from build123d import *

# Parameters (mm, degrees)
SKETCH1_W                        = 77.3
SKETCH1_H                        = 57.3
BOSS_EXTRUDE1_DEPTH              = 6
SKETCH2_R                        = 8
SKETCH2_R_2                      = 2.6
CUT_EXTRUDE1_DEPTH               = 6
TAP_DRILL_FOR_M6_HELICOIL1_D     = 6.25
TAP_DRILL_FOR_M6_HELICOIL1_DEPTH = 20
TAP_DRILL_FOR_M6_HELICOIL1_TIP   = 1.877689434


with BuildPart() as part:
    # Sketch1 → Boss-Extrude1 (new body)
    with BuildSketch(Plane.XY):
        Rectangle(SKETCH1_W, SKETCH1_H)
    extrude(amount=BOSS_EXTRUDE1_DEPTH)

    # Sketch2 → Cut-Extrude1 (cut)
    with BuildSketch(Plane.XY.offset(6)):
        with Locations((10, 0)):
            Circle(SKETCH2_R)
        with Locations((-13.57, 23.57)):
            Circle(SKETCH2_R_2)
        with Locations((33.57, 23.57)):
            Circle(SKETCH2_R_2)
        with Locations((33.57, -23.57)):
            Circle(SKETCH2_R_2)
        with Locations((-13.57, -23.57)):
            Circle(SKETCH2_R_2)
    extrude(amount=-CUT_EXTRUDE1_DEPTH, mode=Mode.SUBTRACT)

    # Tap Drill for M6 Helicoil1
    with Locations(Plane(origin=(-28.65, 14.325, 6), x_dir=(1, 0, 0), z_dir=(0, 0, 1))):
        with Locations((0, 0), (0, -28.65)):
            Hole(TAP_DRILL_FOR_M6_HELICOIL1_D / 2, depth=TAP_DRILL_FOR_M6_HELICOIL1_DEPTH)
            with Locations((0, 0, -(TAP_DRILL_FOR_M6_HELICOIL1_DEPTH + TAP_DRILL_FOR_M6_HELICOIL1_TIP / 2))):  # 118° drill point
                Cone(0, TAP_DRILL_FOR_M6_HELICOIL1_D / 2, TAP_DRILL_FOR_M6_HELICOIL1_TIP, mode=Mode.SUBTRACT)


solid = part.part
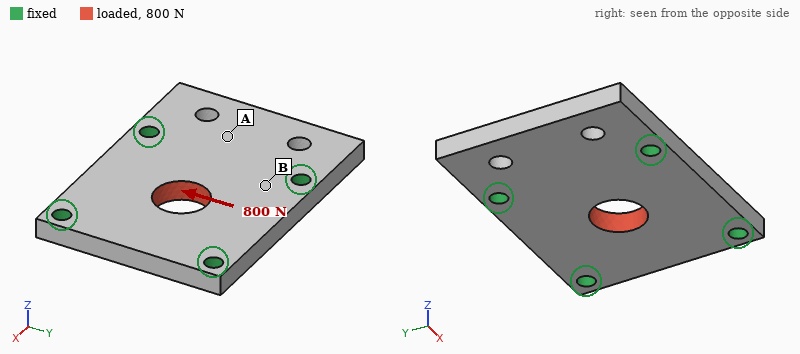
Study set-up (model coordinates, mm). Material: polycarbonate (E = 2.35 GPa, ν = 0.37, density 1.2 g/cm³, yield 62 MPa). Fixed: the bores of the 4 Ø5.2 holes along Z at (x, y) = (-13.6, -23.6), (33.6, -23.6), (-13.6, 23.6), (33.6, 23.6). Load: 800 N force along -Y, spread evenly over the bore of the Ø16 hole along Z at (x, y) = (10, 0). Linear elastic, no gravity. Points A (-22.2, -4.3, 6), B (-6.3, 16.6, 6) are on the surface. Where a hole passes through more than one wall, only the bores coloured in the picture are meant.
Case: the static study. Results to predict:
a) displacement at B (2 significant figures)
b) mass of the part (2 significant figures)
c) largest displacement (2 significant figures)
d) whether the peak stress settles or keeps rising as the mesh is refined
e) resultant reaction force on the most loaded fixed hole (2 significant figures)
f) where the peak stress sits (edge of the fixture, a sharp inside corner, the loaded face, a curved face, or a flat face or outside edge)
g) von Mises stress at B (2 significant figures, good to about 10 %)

14 µm
29 g
40 µm
keeps rising
230 N
edge of the fixture
2.8 MPa
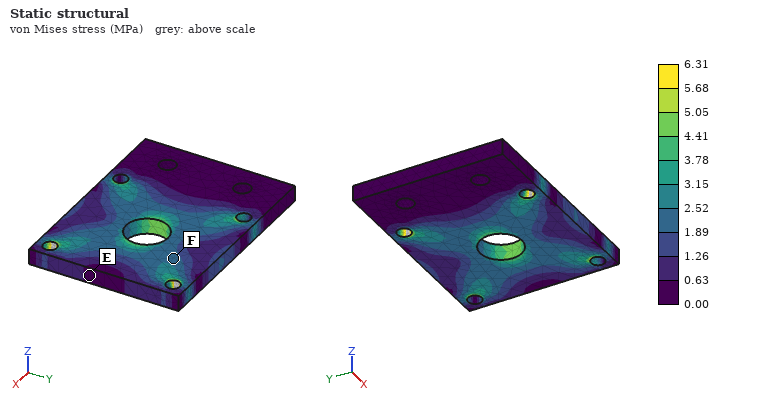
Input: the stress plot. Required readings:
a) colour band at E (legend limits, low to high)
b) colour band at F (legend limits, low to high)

0.00 to 0.63 MPa
1.89 to 2.52 MPa
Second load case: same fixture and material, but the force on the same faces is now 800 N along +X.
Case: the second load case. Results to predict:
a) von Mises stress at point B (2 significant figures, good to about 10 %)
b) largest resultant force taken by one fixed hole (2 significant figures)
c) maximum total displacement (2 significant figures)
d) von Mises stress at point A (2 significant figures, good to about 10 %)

2.4 MPa
230 N
39 µm
0.81 MPa
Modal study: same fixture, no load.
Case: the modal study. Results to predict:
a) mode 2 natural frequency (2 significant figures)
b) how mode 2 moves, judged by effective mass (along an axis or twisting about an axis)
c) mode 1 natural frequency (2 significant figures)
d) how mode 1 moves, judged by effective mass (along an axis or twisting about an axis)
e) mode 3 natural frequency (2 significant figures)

2700 Hz
along Z
1700 Hz
along Z
2900 Hz
